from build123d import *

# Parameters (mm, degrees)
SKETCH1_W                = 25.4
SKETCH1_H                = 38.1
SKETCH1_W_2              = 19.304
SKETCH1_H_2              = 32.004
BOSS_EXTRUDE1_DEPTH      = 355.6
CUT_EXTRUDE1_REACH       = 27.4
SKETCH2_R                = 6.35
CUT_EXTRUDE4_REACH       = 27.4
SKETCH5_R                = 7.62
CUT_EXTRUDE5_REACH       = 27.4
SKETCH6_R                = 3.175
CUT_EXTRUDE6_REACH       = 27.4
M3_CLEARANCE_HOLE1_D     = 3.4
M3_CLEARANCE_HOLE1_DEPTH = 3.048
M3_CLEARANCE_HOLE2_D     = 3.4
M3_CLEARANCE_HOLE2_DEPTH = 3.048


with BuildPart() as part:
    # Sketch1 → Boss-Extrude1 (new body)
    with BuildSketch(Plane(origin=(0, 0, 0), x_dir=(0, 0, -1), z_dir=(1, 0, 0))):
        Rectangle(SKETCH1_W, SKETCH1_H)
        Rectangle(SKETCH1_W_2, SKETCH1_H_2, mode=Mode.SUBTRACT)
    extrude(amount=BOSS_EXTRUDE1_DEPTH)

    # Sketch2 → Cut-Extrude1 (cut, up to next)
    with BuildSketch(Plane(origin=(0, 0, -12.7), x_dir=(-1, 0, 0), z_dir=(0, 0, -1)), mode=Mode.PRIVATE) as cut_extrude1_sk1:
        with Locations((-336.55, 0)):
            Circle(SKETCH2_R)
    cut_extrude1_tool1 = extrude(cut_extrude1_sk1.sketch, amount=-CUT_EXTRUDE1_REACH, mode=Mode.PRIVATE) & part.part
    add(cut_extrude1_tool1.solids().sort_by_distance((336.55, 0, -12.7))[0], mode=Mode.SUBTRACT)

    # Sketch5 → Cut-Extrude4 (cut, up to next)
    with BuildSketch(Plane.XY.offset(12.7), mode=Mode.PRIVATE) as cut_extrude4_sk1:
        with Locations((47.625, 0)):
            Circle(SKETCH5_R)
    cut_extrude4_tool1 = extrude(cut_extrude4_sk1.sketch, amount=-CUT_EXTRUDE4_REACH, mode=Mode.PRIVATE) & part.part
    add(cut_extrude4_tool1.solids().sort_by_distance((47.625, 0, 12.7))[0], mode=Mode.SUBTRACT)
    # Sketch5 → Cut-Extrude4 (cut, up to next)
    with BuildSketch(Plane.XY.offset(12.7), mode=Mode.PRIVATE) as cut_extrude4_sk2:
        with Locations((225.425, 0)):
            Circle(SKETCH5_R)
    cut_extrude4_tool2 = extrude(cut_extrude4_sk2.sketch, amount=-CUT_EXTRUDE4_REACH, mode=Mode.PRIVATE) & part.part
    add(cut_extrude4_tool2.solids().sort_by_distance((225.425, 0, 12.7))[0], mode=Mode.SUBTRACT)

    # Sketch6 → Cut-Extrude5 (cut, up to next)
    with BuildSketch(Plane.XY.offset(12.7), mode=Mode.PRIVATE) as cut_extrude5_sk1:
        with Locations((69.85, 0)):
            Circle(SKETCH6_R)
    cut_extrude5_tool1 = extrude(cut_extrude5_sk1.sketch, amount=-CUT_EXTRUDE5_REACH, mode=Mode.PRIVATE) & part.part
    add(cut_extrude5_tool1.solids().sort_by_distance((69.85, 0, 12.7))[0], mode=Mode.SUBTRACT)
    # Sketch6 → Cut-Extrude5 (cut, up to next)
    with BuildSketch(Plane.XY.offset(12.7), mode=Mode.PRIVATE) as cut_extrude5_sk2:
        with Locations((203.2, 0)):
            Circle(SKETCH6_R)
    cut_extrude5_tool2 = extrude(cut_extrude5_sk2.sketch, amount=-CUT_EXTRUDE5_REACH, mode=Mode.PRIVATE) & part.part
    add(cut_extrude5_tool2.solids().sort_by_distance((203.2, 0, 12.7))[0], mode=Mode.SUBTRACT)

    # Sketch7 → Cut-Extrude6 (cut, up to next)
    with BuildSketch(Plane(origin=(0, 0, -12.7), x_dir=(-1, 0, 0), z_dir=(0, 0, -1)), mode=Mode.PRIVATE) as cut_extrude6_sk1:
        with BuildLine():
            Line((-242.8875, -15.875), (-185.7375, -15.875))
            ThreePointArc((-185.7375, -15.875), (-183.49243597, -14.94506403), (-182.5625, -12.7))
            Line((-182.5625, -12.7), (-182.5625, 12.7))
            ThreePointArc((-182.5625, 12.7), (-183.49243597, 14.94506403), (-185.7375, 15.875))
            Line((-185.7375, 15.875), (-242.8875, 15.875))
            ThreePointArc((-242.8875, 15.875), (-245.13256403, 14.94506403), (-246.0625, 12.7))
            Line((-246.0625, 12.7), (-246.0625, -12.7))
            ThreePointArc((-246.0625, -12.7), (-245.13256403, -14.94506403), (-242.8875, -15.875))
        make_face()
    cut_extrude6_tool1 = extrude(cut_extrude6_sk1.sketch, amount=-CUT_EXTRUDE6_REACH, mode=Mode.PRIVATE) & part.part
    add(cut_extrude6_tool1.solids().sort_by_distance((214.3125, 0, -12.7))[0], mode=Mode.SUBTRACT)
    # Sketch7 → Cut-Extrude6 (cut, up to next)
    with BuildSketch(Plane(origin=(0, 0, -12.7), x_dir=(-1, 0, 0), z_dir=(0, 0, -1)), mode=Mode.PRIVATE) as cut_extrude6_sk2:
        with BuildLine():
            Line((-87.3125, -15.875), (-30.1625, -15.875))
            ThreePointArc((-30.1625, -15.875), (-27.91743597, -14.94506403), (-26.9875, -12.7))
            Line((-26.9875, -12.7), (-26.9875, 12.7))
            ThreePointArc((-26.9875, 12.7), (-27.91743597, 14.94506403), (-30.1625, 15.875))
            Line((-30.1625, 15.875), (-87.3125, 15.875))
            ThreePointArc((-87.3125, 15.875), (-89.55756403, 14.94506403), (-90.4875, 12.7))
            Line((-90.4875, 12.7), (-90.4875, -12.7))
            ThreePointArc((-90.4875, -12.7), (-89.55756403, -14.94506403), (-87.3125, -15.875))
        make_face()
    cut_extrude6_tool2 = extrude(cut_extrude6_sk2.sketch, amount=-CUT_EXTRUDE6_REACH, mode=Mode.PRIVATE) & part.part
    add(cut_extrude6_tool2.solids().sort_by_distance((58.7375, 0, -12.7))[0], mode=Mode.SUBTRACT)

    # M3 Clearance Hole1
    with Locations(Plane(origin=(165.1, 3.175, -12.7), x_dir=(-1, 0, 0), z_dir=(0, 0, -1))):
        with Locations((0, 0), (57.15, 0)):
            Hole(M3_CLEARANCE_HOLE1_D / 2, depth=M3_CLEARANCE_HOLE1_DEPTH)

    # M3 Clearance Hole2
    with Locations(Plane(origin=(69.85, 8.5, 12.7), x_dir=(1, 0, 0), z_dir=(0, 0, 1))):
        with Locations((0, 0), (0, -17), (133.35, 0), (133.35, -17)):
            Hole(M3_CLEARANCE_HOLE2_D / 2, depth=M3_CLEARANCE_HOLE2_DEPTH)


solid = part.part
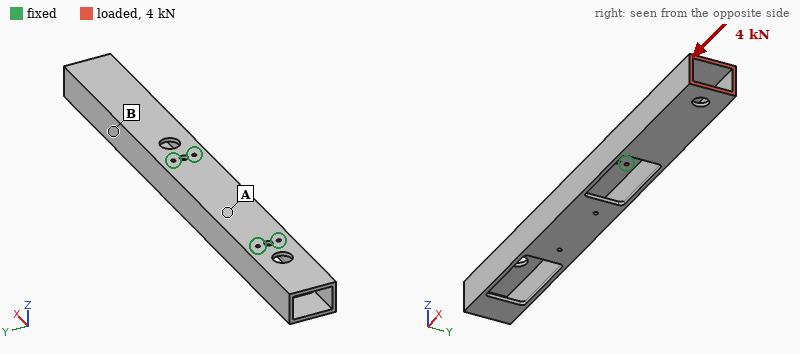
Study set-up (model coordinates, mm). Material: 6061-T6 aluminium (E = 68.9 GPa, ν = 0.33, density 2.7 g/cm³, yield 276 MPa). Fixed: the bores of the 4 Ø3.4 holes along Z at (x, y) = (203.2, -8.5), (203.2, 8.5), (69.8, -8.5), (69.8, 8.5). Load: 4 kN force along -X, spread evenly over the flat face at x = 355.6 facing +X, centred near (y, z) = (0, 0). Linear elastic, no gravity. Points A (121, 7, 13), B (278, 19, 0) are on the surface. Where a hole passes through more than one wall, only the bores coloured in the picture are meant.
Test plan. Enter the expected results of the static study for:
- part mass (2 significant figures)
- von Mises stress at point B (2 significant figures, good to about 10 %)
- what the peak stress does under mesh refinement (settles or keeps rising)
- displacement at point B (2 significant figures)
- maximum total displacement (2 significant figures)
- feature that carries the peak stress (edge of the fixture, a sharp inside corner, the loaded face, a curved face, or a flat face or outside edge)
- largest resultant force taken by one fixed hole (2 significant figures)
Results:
300 g
13 MPa
keeps rising
0.12 mm
0.27 mm
edge of the fixture
1.3 kN
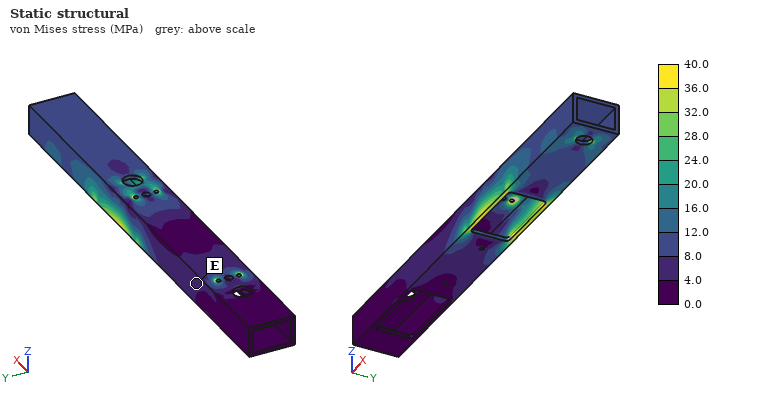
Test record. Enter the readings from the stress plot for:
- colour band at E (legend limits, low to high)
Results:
4.0 to 8.0 MPa
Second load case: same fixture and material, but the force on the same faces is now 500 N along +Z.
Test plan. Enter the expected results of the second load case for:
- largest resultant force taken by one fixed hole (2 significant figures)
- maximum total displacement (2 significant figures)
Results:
1.0 kN
0.88 mm
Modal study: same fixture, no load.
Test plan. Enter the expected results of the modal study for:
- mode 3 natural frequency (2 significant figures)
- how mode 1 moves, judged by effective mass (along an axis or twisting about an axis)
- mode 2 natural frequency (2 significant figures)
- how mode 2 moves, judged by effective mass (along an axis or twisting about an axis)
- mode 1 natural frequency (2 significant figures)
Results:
1500 Hz
along Z
870 Hz
along Y
590 Hz
